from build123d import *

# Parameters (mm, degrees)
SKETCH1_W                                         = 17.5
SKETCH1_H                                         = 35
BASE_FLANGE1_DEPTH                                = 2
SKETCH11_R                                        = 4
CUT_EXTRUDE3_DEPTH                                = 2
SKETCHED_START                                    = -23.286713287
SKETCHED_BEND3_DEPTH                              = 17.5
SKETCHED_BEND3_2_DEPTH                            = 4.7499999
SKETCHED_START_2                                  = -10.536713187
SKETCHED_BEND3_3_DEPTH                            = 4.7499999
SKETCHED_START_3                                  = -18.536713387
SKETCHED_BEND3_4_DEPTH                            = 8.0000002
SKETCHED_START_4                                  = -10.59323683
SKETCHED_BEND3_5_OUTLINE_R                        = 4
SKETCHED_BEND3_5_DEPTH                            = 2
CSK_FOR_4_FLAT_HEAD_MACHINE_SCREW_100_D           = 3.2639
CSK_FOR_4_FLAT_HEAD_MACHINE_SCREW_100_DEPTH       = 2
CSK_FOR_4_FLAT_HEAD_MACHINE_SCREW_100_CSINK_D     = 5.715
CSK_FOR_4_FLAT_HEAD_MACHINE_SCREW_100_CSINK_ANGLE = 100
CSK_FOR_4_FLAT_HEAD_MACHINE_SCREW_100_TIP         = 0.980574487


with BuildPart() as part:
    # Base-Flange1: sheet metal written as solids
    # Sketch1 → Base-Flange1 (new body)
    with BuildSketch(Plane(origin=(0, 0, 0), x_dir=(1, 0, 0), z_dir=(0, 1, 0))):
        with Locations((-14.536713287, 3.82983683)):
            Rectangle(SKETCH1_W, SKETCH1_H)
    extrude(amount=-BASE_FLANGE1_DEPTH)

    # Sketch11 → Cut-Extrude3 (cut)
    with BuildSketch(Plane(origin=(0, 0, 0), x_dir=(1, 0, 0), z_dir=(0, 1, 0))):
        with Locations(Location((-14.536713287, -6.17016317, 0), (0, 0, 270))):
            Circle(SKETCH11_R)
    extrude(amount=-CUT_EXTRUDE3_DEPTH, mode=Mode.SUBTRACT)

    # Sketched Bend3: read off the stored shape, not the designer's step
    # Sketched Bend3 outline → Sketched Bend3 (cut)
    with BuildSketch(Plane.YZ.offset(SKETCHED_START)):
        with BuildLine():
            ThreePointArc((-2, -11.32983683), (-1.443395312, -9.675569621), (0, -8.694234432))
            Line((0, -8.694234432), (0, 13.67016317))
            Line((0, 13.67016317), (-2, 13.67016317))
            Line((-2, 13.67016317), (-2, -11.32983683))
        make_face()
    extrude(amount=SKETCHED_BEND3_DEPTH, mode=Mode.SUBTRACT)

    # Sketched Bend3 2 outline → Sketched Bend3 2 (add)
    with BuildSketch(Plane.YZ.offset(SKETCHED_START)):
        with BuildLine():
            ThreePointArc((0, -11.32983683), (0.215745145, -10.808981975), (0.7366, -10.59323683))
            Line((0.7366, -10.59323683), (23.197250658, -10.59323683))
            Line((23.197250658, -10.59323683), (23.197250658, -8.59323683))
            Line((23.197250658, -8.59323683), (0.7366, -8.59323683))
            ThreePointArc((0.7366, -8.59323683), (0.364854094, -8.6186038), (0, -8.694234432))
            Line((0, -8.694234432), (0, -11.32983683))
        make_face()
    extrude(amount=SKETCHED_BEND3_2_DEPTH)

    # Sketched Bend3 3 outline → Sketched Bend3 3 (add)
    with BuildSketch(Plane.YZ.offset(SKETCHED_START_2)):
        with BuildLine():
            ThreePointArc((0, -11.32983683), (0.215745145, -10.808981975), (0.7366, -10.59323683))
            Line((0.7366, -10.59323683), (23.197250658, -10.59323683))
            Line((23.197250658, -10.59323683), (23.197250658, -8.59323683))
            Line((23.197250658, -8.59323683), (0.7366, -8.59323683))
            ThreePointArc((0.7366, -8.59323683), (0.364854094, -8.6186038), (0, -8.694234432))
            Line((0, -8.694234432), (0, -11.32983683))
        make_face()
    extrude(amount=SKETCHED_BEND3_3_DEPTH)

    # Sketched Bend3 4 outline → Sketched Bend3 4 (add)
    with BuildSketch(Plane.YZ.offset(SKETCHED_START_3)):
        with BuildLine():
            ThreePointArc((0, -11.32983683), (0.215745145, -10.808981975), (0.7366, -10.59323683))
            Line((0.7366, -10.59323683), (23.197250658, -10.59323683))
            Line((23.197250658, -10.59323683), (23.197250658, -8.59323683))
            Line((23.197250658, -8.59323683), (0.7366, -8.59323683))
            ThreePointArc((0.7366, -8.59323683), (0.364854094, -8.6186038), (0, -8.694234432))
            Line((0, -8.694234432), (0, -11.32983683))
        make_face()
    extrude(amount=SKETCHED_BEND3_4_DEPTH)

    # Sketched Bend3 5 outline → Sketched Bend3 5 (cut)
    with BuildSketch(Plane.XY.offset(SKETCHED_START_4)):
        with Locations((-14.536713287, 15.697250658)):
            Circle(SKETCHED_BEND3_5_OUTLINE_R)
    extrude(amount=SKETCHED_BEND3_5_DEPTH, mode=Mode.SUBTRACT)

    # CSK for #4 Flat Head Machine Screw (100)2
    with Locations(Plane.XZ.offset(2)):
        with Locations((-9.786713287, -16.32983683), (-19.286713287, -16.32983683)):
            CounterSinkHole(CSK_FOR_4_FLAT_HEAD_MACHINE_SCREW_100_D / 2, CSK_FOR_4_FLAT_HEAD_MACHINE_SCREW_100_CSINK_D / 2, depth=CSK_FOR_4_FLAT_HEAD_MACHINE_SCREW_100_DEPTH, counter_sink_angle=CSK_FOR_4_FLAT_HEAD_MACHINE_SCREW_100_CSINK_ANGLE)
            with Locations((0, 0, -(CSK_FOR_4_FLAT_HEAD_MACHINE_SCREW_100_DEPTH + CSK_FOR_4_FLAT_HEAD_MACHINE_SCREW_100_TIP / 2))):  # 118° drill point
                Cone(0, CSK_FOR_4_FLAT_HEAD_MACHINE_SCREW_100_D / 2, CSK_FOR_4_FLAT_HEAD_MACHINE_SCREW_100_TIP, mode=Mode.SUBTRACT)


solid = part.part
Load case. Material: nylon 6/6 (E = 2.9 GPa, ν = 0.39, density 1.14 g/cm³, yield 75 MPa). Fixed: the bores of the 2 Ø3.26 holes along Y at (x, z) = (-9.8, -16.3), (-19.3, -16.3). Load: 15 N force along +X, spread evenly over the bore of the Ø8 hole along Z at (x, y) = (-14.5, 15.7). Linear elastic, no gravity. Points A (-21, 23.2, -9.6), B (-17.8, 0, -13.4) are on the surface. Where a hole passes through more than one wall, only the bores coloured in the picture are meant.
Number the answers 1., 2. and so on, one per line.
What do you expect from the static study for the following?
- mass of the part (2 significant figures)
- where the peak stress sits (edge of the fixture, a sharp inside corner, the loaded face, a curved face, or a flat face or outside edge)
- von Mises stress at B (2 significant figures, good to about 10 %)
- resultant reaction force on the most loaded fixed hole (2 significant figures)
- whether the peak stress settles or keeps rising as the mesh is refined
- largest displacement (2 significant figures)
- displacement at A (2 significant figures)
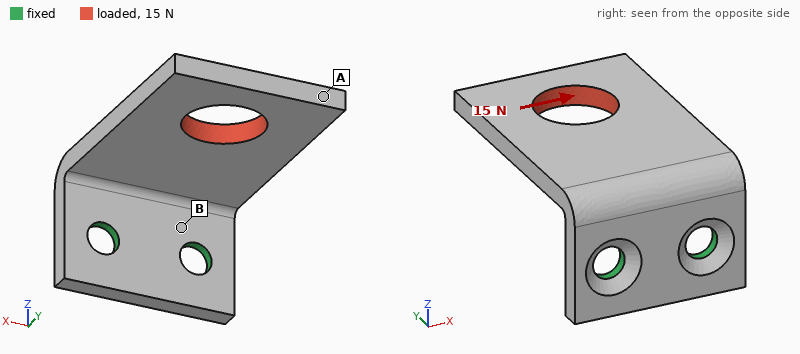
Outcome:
1. 1.2 g
2. edge of the fixture
3. 9.3 MPa
4. 23 N
5. keeps rising
6. 0.38 mm
7. 0.36 mm
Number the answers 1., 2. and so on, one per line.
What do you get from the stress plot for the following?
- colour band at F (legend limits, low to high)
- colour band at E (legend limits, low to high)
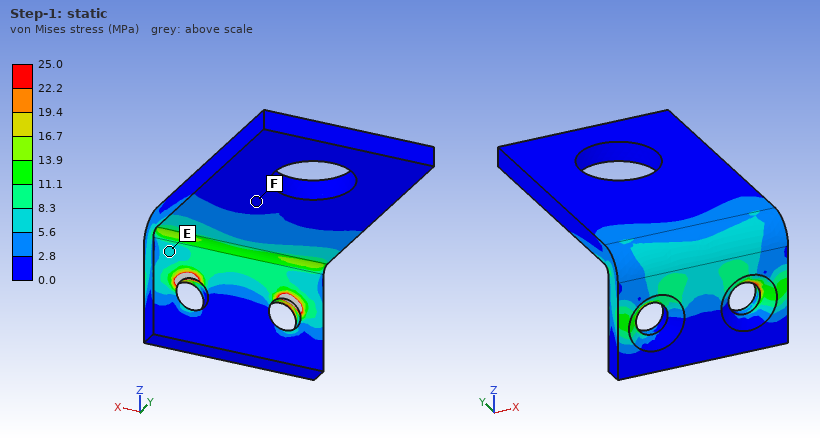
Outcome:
1. 0.0 to 2.8 MPa
2. 5.6 to 8.3 MPa
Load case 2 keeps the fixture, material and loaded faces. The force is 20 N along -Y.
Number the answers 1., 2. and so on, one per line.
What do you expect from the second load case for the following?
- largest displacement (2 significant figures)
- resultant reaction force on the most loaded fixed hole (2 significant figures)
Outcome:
1. 0.39 mm
2. 10 N
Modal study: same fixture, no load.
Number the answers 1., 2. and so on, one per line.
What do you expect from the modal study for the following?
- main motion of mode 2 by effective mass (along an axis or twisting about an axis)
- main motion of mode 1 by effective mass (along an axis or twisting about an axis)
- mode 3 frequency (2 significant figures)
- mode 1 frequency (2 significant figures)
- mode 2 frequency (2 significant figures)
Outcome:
1. along X
2. along Z
3. 2400 Hz
4. 670 Hz
5. 1500 Hz
